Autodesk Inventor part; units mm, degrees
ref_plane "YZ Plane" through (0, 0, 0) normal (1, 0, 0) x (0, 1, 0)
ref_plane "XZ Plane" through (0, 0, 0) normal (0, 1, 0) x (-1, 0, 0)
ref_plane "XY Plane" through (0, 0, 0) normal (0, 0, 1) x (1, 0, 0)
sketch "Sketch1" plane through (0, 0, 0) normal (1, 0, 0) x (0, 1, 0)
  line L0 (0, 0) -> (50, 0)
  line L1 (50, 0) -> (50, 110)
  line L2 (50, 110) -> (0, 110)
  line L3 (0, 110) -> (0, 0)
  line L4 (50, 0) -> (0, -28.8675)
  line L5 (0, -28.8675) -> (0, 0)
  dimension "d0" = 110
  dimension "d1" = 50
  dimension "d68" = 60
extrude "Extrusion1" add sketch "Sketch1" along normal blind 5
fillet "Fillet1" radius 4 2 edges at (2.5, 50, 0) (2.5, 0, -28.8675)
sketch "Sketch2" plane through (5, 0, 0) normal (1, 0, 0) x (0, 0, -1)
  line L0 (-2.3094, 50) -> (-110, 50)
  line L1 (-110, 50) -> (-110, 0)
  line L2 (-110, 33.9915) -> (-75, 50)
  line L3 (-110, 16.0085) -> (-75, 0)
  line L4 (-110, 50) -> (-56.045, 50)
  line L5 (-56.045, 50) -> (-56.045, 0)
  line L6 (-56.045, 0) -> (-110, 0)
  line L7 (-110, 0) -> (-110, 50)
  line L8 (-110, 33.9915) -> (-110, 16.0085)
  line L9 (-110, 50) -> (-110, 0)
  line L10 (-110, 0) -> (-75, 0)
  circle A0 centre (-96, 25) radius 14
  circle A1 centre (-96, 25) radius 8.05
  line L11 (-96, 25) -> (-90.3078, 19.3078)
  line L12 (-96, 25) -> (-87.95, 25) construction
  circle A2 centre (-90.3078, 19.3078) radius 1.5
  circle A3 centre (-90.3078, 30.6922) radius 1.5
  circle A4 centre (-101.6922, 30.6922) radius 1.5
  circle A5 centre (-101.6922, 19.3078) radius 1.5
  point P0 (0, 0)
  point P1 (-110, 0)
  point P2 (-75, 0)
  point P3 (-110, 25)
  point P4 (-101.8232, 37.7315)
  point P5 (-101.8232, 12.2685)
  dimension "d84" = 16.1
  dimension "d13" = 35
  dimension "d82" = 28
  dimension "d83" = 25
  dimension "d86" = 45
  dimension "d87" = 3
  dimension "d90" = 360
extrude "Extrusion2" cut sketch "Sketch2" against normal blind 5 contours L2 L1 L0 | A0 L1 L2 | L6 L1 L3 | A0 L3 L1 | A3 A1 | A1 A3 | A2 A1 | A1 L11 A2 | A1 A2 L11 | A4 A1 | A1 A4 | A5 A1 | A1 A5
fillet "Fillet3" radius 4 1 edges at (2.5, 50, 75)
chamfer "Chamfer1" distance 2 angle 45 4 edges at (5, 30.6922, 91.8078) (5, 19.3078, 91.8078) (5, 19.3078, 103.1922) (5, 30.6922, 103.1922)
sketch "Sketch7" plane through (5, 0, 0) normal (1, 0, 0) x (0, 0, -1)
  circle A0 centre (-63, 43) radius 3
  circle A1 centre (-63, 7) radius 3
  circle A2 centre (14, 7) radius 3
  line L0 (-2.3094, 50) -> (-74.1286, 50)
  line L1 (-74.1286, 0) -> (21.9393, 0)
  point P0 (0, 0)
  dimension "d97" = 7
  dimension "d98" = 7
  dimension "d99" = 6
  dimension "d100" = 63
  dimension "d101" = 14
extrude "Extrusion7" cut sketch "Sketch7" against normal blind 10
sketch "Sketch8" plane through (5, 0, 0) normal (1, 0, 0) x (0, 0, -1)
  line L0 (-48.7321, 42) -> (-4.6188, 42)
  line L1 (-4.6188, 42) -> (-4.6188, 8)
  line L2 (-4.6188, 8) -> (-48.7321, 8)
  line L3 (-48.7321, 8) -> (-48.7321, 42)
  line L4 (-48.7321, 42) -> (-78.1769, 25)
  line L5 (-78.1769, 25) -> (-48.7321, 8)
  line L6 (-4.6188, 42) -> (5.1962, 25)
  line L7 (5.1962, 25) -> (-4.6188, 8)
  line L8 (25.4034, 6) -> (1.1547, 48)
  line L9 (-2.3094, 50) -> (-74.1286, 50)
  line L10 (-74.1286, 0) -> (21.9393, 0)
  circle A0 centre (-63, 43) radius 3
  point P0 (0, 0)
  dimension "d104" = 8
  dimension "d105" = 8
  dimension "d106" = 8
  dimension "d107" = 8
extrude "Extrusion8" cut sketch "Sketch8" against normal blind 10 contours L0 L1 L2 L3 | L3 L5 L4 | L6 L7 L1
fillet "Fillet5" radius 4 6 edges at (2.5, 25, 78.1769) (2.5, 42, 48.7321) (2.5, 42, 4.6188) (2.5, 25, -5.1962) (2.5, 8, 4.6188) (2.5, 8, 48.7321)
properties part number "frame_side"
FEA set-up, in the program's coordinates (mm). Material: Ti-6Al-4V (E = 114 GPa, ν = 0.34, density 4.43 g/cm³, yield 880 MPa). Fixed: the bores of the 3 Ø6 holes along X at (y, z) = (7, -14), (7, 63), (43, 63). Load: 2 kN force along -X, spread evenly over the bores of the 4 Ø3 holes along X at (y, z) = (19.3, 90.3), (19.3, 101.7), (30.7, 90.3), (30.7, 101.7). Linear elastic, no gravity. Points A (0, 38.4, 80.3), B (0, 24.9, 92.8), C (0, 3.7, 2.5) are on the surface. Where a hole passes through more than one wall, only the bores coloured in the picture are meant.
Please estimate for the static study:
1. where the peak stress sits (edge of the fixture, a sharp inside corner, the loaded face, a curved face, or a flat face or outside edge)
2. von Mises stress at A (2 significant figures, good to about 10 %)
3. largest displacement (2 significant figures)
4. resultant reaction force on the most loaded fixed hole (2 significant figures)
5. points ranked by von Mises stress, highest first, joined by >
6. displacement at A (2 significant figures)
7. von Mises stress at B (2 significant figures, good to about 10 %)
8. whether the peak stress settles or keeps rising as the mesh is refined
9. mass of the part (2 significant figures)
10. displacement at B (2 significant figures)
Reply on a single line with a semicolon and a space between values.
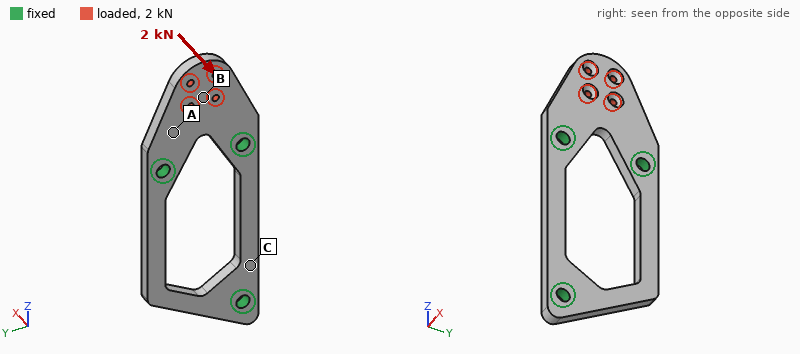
edge of the fixture; 190 MPa; 0.89 mm; 1.0 kN; A > B > C; 0.18 mm; 97 MPa; keeps rising; 74 g; 0.46 mm
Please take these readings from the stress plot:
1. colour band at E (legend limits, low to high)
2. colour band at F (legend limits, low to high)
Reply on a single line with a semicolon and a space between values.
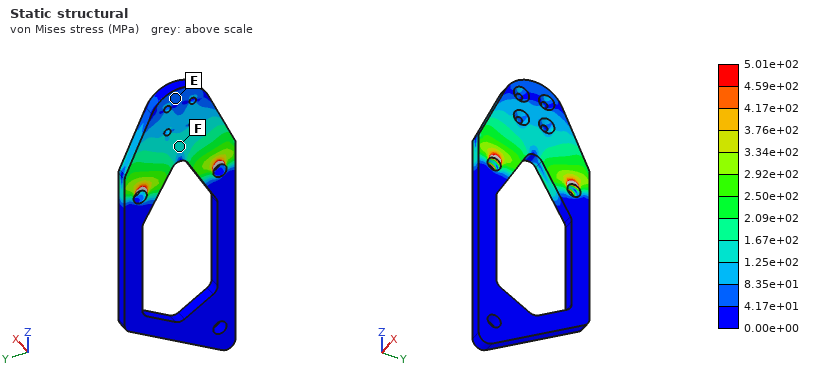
4.17e+01 to 8.35e+01 MPa; 1.25e+02 to 1.67e+02 MPa
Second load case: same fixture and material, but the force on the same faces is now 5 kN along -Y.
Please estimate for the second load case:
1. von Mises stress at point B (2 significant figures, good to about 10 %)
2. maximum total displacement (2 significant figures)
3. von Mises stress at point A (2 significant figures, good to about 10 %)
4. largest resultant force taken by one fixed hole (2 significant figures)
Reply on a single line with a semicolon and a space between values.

49 MPa; 47 µm; 52 MPa; 4.7 kN
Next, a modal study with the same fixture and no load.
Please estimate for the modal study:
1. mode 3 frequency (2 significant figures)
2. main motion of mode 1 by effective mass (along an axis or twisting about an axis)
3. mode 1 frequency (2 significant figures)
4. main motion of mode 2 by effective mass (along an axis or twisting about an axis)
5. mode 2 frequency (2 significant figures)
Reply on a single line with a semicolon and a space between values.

5400 Hz; along X; 2400 Hz; along X; 2700 Hz
